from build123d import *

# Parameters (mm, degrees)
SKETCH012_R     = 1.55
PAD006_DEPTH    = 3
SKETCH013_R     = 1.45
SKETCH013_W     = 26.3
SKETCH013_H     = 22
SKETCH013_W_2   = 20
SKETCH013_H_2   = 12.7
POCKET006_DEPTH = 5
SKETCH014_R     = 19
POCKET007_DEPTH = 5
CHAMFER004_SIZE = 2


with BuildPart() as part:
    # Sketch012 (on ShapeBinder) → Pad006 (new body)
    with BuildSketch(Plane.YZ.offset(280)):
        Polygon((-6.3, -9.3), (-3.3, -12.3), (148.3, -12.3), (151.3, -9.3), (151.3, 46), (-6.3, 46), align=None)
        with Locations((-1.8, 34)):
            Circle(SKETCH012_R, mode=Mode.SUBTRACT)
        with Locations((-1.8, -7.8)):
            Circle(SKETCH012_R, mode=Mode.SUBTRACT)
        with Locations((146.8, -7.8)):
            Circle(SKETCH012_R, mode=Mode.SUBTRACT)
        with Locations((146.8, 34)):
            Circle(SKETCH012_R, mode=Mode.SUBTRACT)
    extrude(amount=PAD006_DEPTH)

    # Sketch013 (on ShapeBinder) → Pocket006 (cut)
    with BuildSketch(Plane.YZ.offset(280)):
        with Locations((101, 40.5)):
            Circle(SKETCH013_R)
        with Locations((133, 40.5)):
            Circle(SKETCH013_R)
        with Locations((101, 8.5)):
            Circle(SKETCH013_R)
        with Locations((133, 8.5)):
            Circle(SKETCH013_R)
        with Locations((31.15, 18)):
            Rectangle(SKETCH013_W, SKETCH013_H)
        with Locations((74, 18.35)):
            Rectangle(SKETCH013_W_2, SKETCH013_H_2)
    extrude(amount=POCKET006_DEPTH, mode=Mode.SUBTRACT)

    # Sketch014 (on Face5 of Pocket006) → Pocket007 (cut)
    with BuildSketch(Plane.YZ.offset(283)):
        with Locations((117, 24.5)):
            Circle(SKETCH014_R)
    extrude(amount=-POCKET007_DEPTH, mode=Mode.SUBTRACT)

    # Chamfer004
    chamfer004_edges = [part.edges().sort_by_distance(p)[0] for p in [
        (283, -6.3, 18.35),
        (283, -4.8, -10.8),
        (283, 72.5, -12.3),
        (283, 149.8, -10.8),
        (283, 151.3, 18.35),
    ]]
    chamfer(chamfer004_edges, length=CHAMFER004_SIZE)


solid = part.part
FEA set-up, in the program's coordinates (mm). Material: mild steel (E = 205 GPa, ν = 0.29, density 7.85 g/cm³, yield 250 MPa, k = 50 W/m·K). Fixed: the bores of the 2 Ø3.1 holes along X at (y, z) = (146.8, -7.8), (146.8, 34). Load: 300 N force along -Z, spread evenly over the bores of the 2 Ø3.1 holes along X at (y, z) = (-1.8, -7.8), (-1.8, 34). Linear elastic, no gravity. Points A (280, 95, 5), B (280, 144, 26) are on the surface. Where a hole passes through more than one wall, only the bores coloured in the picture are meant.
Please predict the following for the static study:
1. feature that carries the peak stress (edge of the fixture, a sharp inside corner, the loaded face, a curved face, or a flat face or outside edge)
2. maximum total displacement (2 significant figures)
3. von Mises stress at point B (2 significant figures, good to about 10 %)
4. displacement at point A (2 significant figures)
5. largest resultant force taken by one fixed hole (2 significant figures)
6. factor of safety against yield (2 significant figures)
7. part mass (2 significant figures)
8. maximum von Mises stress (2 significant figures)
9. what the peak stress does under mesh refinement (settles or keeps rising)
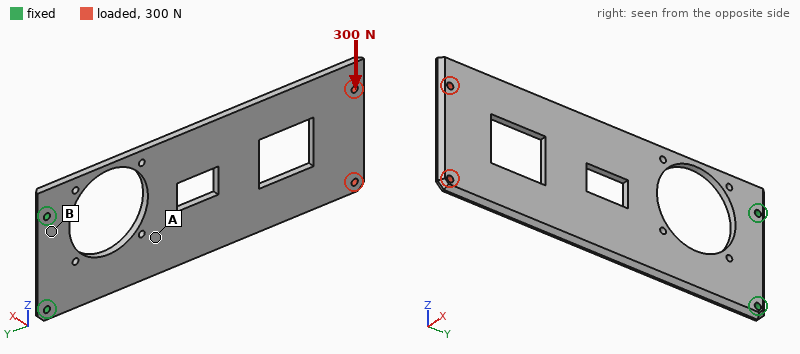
a curved face
0.11 mm
19 MPa
0.024 mm
1.1 kN
1.4
160 g
180 MPa
settles
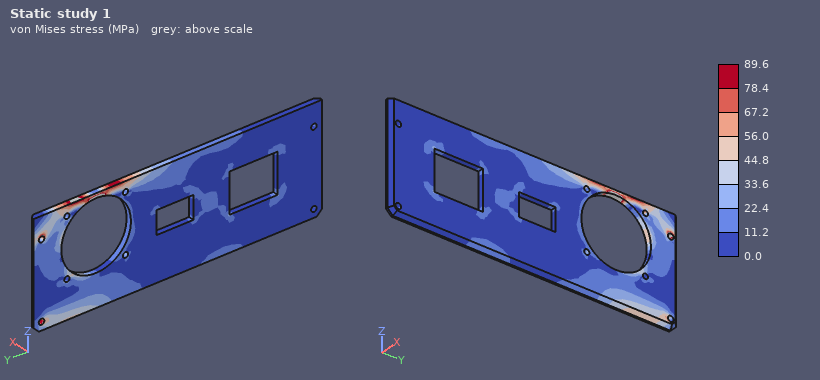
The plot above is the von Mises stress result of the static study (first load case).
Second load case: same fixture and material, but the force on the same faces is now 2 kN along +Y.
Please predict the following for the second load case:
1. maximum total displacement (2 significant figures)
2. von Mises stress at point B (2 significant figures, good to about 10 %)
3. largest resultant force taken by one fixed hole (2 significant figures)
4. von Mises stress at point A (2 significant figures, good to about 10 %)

44 µm
19 MPa
1.0 kN
20 MPa
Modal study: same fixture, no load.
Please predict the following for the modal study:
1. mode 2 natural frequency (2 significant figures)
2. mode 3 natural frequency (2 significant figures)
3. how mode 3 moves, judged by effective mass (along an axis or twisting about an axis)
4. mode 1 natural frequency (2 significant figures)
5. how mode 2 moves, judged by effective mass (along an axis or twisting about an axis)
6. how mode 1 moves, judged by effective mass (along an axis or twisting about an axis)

470 Hz
590 Hz
along X
79 Hz
twisting about Y
along X
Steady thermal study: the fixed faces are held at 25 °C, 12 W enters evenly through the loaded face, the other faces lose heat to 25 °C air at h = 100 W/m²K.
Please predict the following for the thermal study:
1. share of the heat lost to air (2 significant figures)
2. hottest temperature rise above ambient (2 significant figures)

100 %
58 K
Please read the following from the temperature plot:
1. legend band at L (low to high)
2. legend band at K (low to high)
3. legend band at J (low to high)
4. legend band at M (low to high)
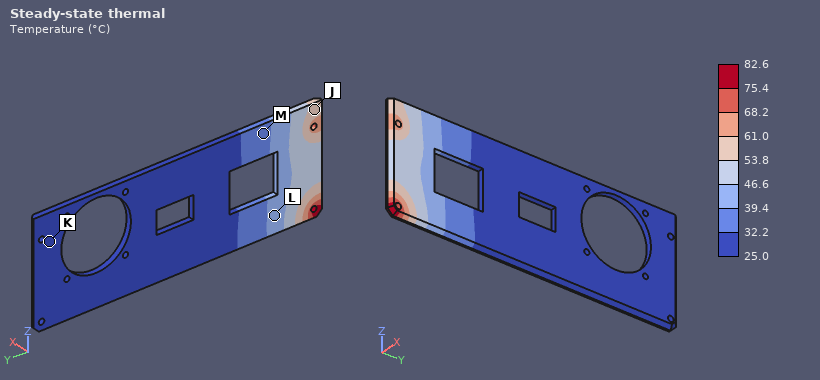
39.4 to 46.6 °C
25.0 to 32.2 °C
53.8 to 61.0 °C
32.2 to 39.4 °C
